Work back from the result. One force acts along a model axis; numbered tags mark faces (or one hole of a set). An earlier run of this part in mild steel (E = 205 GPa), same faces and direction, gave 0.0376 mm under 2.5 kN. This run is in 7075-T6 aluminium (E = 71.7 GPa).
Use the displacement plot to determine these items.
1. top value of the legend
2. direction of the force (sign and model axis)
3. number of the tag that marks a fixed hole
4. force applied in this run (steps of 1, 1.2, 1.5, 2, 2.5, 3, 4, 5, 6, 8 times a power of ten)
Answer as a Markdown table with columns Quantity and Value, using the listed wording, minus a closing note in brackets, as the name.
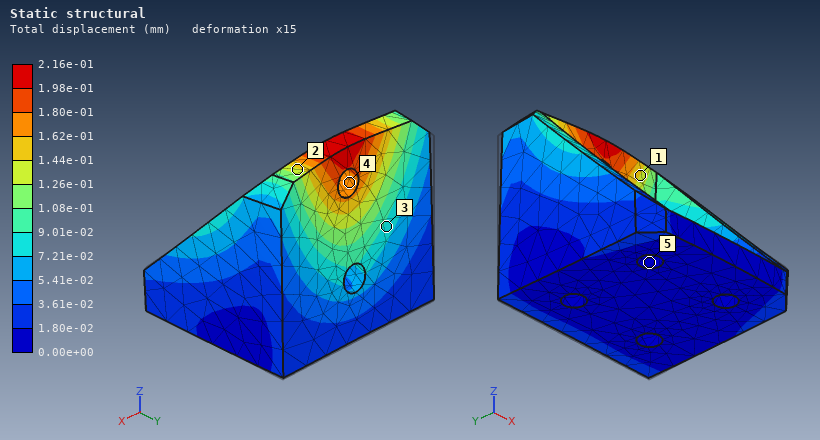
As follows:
| Quantity | Value |
|---|---|
| top value of the legend | 2.16e-01 mm |
| direction of the force | -Y |
| number of the tag that marks a fixed hole | 5 |
| force applied in this run | 5 kN |
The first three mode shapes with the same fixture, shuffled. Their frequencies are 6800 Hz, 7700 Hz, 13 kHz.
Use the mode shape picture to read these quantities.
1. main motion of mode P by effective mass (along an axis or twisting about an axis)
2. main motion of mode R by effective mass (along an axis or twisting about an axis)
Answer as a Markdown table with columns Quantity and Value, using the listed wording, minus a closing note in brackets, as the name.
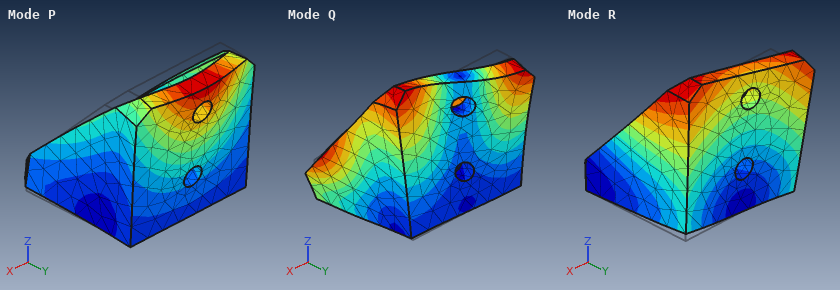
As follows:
| Quantity | Value |
|---|---|
| main motion of mode P by effective mass | along Y |
| main motion of mode R by effective mass | along X |
